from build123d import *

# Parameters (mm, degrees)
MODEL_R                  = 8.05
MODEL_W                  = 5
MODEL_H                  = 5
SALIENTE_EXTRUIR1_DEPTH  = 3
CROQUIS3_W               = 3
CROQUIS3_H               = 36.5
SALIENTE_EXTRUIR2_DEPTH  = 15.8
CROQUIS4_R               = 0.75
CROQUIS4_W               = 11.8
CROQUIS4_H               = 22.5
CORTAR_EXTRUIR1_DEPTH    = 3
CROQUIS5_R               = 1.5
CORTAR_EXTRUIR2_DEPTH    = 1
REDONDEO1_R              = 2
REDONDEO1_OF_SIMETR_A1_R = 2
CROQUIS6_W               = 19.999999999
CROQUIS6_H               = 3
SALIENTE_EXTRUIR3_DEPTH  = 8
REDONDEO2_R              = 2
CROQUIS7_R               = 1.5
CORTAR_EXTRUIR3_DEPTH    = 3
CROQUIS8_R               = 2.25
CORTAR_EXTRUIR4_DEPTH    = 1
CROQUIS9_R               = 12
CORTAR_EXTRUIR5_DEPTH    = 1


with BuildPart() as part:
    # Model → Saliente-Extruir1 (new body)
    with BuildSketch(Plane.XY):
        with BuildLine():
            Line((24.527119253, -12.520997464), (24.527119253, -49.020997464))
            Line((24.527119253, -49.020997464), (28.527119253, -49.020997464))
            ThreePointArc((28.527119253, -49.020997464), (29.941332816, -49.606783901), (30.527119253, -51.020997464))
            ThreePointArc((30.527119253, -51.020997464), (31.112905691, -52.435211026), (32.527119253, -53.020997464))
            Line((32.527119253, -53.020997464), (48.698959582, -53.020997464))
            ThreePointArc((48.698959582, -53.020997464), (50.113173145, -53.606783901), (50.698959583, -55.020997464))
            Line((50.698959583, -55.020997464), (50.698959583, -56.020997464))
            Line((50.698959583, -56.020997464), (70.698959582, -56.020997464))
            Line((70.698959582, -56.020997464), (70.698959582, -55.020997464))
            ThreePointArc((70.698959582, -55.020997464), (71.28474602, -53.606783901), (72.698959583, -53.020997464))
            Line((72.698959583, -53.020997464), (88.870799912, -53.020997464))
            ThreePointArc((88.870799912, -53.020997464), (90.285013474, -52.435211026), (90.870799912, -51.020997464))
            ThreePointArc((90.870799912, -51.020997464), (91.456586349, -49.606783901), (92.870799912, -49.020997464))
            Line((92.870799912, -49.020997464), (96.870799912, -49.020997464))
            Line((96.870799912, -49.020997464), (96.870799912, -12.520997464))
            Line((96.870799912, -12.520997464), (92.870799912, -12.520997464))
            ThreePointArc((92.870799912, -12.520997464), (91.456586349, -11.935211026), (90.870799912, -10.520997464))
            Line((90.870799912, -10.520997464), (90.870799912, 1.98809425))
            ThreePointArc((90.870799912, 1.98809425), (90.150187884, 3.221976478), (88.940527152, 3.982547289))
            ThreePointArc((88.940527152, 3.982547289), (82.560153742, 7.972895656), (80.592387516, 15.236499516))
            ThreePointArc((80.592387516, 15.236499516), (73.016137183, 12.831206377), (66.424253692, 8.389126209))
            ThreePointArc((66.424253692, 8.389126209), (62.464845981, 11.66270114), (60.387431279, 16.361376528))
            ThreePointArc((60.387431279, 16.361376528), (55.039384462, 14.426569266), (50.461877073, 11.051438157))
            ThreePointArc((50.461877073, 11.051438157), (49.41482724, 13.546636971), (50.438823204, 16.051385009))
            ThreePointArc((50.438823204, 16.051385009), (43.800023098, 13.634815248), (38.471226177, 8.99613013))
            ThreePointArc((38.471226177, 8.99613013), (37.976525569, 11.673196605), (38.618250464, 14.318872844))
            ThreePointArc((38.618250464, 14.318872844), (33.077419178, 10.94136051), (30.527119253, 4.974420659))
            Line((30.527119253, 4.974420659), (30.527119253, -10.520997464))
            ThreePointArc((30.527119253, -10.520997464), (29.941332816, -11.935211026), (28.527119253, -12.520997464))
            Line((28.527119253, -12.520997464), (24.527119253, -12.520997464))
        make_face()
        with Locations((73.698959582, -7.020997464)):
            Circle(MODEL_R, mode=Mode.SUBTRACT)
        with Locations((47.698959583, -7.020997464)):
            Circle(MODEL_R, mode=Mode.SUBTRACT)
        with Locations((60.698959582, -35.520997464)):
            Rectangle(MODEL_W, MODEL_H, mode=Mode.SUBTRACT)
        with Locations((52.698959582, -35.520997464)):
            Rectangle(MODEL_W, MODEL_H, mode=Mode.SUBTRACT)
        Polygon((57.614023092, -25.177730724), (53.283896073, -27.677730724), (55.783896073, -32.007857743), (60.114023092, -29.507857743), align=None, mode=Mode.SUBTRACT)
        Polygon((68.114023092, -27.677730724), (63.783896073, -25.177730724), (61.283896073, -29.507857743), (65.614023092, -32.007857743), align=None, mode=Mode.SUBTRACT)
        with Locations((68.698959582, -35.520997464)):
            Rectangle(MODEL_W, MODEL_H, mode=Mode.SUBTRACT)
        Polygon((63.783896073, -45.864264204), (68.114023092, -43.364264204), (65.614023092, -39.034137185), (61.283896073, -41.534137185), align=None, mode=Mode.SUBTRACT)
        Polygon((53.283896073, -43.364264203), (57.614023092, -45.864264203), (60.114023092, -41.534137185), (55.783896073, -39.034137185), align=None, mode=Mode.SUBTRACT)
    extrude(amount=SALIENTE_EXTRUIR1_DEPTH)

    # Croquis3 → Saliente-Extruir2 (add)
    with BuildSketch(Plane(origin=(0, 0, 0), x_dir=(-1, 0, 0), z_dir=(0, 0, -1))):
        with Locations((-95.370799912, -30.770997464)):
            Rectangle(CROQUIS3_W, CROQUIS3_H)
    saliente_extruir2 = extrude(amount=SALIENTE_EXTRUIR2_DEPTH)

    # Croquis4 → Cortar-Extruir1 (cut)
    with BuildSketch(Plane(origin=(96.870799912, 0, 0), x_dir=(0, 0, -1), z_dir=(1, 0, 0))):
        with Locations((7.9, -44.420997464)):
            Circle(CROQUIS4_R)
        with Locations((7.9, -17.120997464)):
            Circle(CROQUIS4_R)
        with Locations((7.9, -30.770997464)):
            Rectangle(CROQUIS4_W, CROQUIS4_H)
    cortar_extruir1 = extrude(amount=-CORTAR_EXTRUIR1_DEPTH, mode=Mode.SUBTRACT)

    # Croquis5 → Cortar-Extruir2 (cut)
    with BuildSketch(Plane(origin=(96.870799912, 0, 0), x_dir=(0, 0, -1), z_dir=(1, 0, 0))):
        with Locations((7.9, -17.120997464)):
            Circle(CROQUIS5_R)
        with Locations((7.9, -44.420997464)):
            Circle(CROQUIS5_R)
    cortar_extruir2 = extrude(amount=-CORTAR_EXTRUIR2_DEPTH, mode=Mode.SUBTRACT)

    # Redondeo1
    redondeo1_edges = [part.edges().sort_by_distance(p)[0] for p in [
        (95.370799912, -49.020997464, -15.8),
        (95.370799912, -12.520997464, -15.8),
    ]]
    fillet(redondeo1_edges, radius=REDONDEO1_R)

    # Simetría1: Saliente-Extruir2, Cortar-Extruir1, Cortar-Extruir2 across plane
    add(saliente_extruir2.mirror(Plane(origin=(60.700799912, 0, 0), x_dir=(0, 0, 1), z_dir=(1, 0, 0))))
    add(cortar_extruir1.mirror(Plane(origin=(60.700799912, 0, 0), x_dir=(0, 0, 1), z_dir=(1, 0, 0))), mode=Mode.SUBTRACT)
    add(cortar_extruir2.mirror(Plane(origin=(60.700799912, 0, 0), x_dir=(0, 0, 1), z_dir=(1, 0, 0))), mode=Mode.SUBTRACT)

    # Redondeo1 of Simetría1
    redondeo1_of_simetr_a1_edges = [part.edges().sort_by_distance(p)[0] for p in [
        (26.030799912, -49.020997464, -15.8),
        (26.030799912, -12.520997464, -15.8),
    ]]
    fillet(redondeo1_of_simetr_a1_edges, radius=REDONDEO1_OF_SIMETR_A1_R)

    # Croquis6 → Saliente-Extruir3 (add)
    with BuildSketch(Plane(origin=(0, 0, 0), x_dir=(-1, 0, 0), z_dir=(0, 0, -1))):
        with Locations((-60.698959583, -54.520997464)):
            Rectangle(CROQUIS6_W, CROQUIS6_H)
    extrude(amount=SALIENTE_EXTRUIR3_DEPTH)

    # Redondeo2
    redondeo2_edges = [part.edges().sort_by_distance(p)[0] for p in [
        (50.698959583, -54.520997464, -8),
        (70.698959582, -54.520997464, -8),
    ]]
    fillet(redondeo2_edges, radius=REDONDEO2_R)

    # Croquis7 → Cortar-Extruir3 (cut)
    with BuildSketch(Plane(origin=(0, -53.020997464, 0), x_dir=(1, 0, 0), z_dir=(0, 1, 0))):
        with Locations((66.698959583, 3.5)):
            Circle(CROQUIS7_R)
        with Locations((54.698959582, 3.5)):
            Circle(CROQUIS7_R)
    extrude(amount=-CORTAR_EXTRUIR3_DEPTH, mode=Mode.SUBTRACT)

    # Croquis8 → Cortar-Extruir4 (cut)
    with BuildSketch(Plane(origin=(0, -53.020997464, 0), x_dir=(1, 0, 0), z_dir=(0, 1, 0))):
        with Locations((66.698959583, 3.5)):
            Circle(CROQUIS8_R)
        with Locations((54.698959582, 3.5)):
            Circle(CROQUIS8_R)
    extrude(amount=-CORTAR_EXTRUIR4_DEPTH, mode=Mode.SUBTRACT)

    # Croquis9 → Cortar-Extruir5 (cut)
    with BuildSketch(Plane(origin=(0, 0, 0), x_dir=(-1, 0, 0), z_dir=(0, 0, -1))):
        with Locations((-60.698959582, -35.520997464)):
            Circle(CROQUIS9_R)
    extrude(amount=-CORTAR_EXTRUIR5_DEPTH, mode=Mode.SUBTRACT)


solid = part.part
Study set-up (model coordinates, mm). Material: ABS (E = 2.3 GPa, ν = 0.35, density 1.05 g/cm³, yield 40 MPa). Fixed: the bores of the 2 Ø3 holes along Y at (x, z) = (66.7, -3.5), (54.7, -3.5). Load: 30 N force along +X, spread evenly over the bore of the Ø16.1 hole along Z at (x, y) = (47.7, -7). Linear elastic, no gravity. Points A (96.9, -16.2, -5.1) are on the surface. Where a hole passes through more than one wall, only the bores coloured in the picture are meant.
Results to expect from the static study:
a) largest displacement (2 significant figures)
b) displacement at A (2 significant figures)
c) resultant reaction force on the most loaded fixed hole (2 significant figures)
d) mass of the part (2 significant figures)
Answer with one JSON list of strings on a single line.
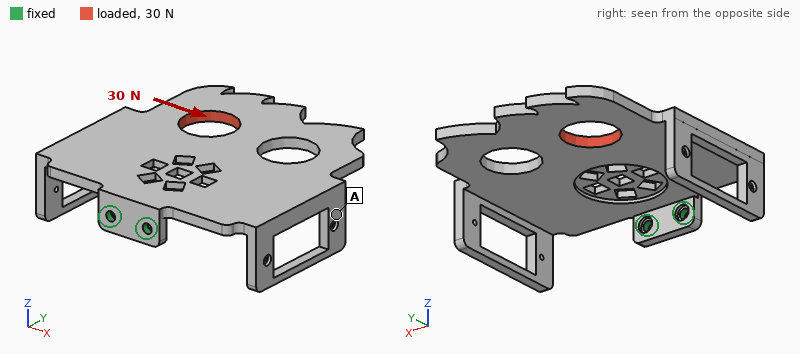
["1.2 mm", "1.0 mm", "110 N", "14 g"]
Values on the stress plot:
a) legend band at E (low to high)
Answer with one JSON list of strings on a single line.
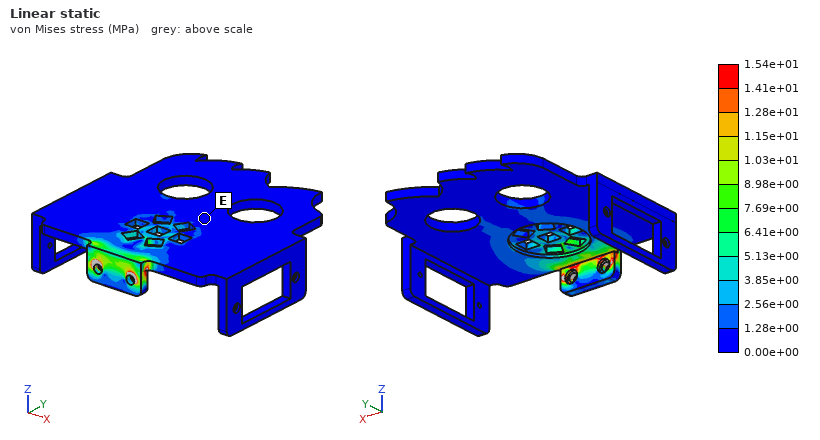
["0.00e+00 to 1.28e+00 MPa"]
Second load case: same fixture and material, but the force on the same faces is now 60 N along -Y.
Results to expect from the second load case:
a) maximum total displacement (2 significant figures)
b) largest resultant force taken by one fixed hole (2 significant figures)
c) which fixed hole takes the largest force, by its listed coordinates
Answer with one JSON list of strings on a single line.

["1.1 mm", "87 N", "(54.7, -3.5)"]
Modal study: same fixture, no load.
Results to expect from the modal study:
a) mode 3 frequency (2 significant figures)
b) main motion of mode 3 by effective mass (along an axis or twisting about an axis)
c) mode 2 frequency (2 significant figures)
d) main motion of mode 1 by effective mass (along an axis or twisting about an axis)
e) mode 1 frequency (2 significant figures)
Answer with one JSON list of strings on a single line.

["330 Hz", "along X", "190 Hz", "along Z", "97 Hz"]
